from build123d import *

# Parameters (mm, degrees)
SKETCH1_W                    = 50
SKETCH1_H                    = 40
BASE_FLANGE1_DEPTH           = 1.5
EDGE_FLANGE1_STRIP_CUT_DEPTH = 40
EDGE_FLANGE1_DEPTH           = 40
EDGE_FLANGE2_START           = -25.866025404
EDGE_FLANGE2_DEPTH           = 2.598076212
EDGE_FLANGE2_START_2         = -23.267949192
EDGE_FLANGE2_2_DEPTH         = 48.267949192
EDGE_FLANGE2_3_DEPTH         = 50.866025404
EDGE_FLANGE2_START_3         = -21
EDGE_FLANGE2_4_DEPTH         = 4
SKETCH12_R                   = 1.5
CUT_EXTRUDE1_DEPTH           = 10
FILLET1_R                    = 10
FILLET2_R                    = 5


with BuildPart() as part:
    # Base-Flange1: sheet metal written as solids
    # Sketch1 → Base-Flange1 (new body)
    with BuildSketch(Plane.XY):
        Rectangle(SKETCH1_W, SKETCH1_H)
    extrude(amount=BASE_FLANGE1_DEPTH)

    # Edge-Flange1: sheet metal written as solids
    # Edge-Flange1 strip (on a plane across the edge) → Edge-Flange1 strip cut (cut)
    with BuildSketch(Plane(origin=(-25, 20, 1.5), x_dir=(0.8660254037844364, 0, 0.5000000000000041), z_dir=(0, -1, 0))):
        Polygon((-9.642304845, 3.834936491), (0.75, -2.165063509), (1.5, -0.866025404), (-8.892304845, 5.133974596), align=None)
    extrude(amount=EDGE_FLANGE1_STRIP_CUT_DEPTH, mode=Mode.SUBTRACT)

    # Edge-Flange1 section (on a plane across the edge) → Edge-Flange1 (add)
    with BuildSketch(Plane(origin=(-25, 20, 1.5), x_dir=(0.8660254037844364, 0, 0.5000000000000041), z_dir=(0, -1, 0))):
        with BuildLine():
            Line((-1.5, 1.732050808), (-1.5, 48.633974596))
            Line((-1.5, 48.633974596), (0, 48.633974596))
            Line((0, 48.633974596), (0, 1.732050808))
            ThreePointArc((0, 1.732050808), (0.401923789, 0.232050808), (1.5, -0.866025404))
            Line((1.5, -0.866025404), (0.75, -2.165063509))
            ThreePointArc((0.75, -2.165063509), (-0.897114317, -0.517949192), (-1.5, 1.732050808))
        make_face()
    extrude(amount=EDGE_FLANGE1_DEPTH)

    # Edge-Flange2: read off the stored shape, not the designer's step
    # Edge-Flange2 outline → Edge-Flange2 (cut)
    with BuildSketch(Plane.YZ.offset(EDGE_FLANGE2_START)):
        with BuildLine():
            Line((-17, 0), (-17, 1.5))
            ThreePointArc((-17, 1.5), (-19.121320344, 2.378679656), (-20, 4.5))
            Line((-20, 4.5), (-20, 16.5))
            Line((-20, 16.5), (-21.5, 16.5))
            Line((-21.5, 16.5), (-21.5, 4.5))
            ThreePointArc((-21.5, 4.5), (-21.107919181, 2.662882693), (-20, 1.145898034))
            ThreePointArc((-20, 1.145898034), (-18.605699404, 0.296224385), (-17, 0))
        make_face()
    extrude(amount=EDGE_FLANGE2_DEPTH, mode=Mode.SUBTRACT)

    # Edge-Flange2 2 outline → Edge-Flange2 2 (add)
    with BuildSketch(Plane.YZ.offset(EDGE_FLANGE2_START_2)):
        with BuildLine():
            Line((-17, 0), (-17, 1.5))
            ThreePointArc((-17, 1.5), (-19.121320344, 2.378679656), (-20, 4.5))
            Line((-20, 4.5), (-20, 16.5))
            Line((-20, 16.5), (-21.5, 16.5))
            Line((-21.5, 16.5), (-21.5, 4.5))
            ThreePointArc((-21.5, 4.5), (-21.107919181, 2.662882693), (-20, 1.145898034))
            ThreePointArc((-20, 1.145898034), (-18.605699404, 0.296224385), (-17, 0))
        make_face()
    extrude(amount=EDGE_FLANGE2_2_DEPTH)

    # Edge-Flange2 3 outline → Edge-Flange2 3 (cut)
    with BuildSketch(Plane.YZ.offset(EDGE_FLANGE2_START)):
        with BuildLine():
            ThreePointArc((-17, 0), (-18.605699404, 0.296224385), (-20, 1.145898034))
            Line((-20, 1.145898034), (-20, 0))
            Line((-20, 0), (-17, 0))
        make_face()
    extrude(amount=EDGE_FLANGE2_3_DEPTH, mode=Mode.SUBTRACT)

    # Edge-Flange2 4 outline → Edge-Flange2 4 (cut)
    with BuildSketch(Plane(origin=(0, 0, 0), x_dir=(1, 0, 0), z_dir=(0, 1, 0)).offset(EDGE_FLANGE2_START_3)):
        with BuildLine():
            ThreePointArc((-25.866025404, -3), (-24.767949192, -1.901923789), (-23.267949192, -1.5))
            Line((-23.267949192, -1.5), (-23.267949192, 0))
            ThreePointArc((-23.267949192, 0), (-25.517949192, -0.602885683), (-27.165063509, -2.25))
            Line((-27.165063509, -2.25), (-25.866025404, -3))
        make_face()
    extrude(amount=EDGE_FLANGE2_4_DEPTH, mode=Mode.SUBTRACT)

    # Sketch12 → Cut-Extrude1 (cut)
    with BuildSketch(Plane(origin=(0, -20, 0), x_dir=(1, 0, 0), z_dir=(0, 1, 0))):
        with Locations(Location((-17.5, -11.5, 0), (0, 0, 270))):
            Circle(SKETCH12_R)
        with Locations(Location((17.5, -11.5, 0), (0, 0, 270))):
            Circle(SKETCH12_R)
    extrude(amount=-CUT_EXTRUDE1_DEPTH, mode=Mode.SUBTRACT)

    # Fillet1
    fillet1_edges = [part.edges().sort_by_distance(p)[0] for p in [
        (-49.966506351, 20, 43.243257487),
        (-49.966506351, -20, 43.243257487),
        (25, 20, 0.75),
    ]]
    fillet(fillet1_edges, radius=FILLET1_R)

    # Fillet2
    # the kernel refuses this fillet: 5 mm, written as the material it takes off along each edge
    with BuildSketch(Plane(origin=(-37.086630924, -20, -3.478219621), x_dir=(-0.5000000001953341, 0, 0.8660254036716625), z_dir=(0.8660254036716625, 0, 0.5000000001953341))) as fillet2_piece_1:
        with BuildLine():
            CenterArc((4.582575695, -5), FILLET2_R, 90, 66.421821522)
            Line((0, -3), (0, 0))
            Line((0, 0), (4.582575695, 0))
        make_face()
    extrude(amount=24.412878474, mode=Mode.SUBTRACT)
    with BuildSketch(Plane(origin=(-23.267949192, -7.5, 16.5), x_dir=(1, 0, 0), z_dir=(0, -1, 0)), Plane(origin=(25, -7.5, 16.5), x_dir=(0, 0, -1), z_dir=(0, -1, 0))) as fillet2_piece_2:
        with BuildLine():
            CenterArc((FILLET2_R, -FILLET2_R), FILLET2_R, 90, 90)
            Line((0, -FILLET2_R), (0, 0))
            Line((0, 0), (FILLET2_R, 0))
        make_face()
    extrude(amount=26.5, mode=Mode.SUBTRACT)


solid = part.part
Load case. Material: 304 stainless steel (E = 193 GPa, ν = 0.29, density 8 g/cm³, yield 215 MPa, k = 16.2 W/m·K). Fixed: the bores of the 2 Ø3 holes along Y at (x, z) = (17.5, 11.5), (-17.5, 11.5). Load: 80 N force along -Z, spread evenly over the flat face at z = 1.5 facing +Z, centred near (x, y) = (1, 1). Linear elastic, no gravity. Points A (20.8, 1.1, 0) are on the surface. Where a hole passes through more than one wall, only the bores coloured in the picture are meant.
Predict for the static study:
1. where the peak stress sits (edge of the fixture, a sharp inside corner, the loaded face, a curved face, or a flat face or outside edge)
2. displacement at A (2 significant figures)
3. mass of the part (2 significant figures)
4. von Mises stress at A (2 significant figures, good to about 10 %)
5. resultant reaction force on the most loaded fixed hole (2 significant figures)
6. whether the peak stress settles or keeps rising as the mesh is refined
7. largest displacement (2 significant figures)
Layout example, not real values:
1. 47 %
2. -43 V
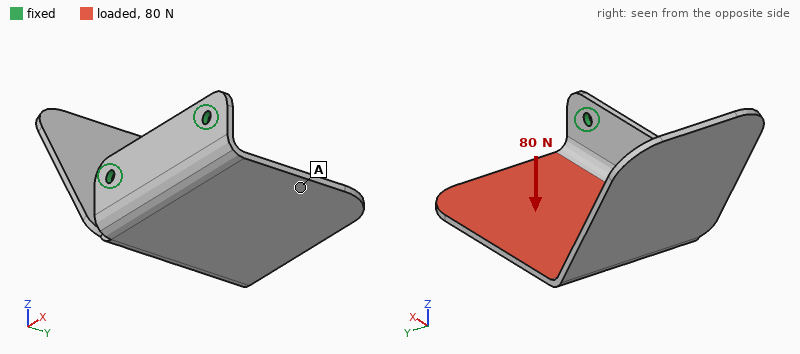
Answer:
1. edge of the fixture
2. 0.25 mm
3. 55 g
4. 17 MPa
5. 45 N
6. keeps rising
7. 0.65 mm
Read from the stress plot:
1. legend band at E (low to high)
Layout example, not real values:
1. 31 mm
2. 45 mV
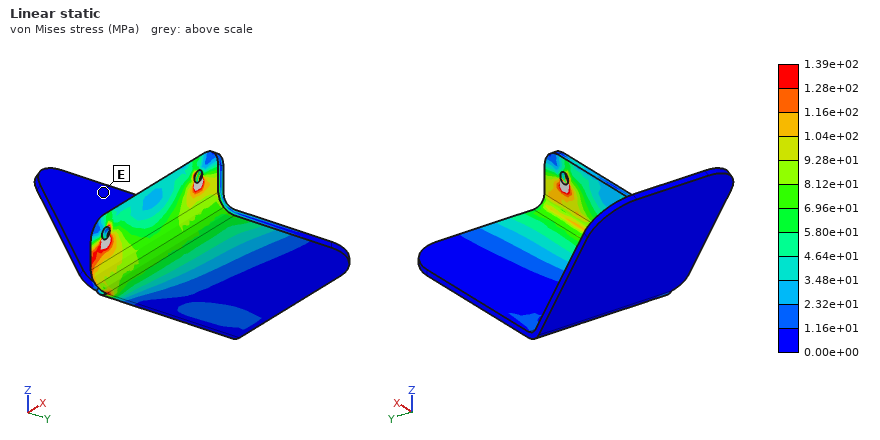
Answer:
1. 0.00e+00 to 1.16e+01 MPa
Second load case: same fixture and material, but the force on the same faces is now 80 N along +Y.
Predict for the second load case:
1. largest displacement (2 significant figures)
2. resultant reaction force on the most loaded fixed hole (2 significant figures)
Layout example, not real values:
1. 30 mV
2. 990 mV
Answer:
1. 83 µm
2. 41 N
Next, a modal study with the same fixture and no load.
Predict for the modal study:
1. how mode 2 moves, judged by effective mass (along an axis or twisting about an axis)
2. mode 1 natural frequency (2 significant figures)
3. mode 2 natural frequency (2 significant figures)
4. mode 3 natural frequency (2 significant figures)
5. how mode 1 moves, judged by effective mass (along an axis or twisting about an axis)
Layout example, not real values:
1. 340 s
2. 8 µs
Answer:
1. along X
2. 240 Hz
3. 380 Hz
4. 970 Hz
5. along Z
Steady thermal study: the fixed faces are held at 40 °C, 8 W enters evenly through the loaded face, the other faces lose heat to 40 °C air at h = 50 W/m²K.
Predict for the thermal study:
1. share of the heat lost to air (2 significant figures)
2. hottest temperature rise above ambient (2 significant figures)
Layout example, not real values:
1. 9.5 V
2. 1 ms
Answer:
1. 84 %
2. 58 K
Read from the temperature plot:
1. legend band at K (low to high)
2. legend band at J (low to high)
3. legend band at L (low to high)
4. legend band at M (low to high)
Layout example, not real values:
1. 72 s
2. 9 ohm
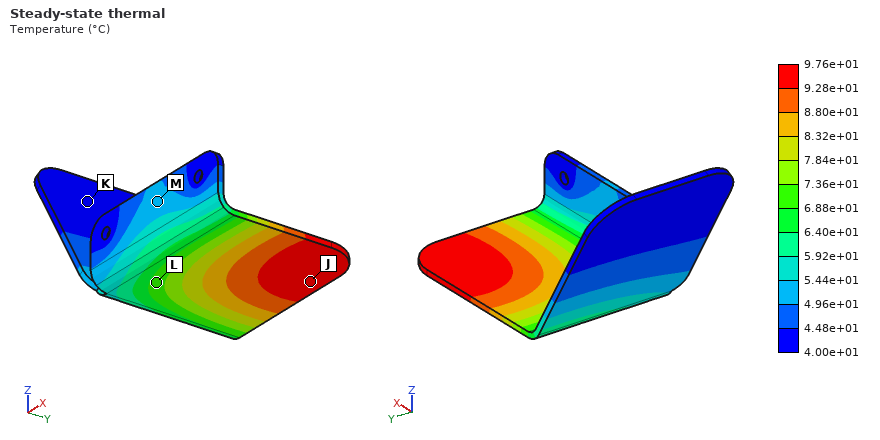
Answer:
1. 4.00e+01 to 4.48e+01 °C
2. 9.28e+01 to 9.76e+01 °C
3. 6.88e+01 to 7.36e+01 °C
4. 4.96e+01 to 5.44e+01 °C
